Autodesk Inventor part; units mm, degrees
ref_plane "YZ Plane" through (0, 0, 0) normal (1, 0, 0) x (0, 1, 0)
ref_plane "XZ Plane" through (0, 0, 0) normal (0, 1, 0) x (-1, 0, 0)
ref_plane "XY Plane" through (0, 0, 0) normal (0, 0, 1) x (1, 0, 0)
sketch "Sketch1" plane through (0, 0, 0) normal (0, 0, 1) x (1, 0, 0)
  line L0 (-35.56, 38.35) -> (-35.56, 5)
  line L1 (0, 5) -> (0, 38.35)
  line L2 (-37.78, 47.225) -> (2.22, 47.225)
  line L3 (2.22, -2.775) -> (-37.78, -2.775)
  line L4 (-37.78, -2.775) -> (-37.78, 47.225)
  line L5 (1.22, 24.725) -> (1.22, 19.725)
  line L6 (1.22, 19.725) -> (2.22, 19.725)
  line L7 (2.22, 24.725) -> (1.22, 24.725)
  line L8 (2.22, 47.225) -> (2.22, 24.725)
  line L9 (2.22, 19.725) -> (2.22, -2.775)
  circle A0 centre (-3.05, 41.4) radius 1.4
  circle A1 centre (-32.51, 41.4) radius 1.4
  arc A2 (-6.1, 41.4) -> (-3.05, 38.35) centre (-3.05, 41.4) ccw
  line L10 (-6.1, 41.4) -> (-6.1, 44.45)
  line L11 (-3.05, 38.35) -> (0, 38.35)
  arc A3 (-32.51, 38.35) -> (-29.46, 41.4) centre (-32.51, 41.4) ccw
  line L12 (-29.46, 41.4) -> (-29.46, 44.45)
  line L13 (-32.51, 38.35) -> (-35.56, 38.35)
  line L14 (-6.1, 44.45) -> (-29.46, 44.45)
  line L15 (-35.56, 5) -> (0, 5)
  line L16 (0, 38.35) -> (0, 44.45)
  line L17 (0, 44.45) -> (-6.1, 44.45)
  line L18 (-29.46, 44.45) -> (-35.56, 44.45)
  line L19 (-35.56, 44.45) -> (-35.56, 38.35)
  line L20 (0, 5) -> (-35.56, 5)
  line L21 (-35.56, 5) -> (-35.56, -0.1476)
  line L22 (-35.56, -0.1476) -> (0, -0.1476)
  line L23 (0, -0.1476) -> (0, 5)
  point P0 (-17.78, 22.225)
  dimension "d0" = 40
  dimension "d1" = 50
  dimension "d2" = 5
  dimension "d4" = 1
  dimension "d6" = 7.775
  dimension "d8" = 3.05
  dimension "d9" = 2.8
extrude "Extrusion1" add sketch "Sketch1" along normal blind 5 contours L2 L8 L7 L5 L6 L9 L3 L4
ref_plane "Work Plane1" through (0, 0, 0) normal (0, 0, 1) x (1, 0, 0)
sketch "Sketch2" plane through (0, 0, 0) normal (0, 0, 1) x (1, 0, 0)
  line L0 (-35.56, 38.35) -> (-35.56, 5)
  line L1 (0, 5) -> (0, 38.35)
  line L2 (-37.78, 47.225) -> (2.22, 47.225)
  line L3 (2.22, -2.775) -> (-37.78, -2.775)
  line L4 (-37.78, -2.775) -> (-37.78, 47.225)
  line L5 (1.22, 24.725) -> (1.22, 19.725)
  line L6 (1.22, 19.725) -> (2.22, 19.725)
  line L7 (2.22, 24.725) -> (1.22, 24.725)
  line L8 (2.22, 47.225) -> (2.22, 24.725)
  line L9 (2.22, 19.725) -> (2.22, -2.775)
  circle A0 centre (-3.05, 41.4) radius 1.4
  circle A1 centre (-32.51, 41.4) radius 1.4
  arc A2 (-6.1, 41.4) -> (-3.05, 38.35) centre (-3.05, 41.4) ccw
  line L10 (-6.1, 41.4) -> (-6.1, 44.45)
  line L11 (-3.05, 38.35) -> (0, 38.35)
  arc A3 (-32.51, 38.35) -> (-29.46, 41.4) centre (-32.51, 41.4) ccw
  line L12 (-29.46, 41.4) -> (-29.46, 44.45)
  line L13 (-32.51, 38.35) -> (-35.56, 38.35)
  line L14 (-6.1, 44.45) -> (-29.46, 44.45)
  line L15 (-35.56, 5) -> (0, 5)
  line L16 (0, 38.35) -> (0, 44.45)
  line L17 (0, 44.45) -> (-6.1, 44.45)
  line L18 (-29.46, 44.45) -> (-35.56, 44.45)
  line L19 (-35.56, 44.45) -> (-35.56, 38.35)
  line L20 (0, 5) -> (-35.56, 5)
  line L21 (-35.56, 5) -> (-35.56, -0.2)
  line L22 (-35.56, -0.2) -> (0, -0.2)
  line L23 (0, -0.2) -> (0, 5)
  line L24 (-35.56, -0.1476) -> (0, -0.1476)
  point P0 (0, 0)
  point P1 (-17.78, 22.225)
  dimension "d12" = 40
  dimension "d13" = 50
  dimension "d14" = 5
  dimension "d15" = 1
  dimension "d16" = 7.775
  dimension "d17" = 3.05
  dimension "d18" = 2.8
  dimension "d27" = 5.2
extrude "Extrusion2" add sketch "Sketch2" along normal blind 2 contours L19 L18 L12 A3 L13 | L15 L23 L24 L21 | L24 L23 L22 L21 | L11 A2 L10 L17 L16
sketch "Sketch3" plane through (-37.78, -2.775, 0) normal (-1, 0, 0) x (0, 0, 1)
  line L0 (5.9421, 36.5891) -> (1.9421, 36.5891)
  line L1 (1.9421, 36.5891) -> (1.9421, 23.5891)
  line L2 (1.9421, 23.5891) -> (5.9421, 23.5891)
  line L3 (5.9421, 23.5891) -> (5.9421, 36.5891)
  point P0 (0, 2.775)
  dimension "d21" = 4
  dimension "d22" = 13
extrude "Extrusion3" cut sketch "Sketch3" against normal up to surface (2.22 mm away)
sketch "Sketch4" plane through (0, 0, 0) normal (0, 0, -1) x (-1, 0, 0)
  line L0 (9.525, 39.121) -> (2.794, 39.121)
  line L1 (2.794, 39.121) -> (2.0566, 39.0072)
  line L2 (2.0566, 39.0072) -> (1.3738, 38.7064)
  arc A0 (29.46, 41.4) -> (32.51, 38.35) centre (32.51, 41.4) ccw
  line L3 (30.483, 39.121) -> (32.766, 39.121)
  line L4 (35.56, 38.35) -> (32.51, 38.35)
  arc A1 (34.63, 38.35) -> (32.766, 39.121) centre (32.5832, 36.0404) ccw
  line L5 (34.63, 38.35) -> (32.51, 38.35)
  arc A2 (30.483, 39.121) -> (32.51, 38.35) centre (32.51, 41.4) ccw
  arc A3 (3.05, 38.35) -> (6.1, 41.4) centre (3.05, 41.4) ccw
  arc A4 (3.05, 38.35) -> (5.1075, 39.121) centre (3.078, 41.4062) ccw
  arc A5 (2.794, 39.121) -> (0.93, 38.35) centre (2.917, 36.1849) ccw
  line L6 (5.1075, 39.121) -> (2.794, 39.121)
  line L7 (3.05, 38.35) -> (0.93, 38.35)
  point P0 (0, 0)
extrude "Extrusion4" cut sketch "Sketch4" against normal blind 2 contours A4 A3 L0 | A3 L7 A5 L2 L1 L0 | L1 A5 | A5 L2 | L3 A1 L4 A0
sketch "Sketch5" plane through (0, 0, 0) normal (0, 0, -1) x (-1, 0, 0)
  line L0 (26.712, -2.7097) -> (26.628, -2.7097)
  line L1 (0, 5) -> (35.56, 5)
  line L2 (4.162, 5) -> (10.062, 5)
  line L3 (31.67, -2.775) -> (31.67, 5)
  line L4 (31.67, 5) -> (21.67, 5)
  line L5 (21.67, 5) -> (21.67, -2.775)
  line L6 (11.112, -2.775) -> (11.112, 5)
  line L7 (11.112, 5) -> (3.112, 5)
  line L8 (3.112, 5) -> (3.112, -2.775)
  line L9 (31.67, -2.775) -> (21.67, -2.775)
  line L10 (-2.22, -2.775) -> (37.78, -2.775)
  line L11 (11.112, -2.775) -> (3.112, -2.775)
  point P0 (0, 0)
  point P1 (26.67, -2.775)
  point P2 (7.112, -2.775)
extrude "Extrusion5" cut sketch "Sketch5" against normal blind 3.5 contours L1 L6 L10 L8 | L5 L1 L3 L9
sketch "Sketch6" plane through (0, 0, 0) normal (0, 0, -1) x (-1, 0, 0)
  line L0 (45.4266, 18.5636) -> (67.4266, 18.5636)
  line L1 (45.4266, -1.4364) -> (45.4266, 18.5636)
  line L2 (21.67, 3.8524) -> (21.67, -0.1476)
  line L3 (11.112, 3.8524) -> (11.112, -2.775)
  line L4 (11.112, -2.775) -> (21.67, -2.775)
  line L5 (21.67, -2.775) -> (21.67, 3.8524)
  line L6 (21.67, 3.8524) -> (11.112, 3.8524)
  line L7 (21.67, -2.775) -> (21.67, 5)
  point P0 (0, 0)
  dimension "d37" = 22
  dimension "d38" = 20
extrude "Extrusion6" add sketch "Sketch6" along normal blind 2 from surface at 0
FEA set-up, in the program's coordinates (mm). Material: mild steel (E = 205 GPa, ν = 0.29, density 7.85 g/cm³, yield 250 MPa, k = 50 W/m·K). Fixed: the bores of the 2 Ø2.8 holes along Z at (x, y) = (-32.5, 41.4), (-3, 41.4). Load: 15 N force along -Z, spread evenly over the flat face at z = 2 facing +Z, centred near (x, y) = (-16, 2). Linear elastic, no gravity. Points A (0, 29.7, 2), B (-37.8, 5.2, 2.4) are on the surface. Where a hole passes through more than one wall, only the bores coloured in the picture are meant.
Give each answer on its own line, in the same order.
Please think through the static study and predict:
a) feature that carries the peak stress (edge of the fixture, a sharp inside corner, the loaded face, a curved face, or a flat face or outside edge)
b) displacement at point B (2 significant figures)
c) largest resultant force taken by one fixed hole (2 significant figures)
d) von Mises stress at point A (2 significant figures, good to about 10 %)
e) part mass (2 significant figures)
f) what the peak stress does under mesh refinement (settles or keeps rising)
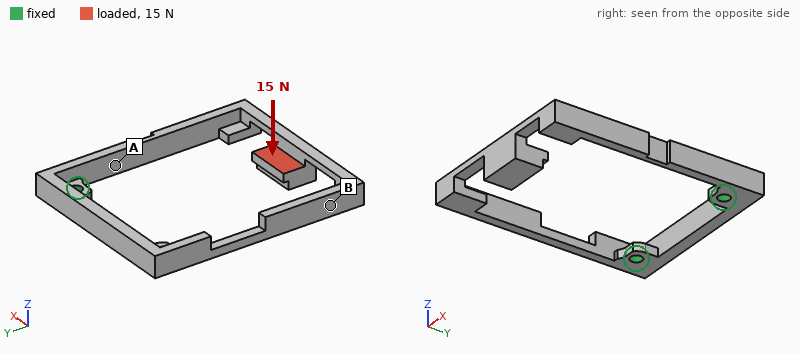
edge of the fixture
0.14 mm
12 N
23 MPa
17 g
keeps rising
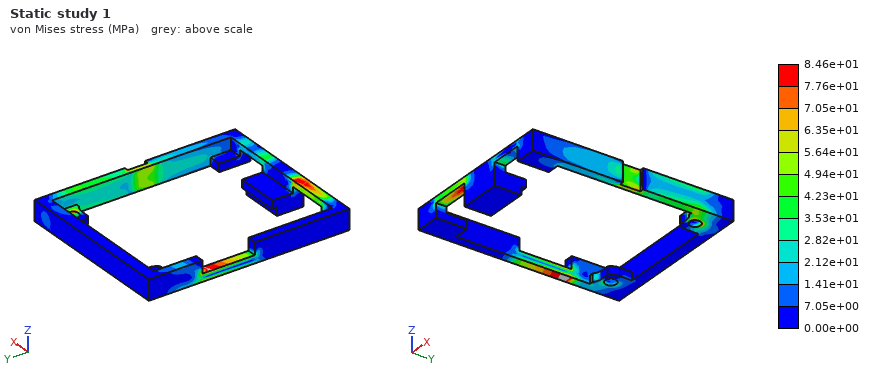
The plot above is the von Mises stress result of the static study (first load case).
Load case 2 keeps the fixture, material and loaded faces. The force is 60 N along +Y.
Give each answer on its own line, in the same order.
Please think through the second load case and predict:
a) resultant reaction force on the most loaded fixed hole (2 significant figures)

40 N
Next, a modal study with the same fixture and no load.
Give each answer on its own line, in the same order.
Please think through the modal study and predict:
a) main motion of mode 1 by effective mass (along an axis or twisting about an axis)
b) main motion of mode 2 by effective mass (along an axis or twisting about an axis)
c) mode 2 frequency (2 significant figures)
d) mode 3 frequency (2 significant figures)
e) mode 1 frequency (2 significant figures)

along Z
along X
810 Hz
1300 Hz
580 Hz
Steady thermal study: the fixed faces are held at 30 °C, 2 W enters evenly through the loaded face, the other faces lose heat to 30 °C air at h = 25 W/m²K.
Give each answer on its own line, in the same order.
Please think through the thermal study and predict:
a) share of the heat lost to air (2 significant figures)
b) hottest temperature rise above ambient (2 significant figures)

74 %
78 K
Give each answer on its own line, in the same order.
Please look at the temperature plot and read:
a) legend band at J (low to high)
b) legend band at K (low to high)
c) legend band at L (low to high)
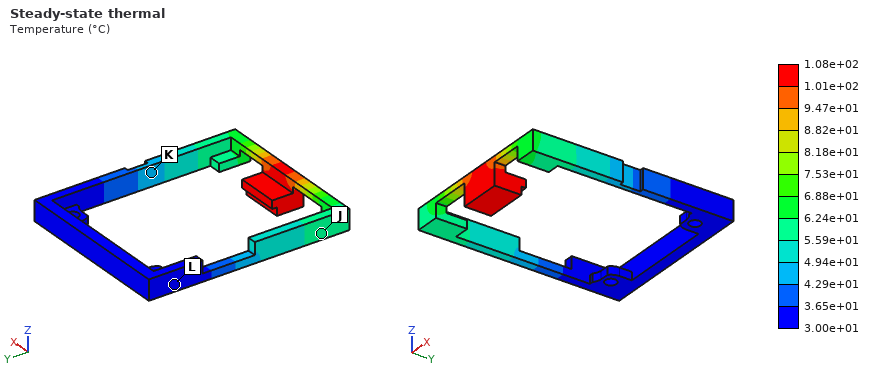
5.59e+01 to 6.24e+01 °C
4.29e+01 to 4.94e+01 °C
3.00e+01 to 3.65e+01 °C
